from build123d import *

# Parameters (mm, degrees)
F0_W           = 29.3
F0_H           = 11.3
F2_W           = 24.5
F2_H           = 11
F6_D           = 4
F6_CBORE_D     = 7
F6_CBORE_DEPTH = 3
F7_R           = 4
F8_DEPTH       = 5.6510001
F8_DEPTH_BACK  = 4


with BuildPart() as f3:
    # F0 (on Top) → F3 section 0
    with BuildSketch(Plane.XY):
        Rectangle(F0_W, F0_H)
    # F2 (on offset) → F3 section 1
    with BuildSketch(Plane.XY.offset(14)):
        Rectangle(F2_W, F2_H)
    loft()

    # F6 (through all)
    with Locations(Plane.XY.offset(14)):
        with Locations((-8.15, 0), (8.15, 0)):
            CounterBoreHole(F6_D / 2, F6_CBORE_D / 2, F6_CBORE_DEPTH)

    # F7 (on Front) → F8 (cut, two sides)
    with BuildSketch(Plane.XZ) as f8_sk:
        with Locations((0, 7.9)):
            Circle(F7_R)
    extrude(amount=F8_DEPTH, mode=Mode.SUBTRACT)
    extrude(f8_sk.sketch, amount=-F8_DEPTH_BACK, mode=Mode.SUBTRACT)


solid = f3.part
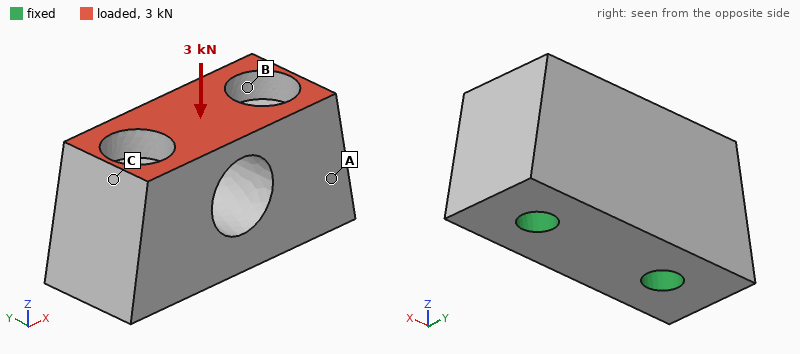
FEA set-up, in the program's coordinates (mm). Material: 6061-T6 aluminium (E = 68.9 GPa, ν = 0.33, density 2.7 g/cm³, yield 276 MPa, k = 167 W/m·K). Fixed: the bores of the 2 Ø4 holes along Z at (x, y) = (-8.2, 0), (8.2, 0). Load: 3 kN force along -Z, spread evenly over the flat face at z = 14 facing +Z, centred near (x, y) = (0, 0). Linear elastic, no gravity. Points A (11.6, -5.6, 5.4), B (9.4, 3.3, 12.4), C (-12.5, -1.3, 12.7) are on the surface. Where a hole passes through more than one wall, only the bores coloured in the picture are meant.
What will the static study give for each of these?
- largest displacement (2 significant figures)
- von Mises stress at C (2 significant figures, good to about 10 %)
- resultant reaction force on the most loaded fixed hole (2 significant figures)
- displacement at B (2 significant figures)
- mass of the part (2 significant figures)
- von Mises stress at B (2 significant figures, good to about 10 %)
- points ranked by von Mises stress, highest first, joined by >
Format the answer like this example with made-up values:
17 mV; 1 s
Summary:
7.3 µm; 11 MPa; 1.6 kN; 1.4 µm; 8.7 g; 18 MPa; B > C > A
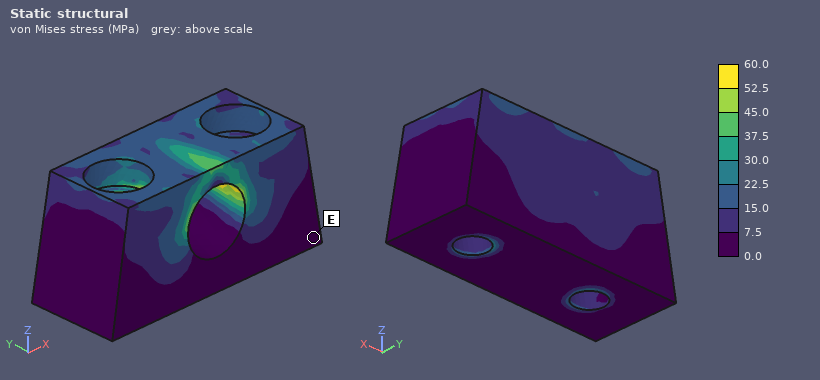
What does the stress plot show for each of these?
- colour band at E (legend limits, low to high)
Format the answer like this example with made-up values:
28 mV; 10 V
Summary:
0.0 to 7.5 MPa
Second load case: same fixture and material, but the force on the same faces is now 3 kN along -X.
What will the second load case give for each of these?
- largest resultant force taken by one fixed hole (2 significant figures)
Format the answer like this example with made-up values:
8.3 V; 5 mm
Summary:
1.7 kN
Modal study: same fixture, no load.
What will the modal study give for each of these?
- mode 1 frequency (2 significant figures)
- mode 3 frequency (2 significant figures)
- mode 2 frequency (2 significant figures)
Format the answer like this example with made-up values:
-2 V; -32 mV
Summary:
66 kHz; 89 kHz; 84 kHz
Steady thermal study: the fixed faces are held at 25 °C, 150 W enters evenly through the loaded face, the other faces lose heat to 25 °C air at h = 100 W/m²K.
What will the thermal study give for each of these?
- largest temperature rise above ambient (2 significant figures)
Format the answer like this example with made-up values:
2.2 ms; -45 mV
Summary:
51 K
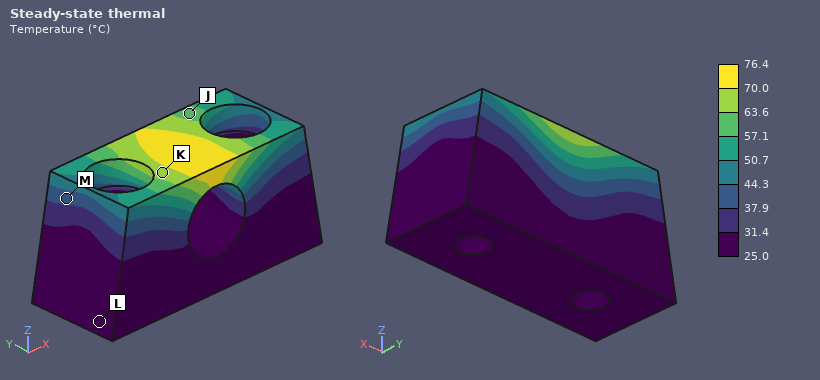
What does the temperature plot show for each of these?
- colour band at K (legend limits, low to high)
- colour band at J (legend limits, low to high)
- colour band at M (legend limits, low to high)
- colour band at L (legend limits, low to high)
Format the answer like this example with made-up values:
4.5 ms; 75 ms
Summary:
63.6 to 70.0 °C; 57.1 to 63.6 °C; 37.9 to 44.3 °C; 25.0 to 31.4 °C
